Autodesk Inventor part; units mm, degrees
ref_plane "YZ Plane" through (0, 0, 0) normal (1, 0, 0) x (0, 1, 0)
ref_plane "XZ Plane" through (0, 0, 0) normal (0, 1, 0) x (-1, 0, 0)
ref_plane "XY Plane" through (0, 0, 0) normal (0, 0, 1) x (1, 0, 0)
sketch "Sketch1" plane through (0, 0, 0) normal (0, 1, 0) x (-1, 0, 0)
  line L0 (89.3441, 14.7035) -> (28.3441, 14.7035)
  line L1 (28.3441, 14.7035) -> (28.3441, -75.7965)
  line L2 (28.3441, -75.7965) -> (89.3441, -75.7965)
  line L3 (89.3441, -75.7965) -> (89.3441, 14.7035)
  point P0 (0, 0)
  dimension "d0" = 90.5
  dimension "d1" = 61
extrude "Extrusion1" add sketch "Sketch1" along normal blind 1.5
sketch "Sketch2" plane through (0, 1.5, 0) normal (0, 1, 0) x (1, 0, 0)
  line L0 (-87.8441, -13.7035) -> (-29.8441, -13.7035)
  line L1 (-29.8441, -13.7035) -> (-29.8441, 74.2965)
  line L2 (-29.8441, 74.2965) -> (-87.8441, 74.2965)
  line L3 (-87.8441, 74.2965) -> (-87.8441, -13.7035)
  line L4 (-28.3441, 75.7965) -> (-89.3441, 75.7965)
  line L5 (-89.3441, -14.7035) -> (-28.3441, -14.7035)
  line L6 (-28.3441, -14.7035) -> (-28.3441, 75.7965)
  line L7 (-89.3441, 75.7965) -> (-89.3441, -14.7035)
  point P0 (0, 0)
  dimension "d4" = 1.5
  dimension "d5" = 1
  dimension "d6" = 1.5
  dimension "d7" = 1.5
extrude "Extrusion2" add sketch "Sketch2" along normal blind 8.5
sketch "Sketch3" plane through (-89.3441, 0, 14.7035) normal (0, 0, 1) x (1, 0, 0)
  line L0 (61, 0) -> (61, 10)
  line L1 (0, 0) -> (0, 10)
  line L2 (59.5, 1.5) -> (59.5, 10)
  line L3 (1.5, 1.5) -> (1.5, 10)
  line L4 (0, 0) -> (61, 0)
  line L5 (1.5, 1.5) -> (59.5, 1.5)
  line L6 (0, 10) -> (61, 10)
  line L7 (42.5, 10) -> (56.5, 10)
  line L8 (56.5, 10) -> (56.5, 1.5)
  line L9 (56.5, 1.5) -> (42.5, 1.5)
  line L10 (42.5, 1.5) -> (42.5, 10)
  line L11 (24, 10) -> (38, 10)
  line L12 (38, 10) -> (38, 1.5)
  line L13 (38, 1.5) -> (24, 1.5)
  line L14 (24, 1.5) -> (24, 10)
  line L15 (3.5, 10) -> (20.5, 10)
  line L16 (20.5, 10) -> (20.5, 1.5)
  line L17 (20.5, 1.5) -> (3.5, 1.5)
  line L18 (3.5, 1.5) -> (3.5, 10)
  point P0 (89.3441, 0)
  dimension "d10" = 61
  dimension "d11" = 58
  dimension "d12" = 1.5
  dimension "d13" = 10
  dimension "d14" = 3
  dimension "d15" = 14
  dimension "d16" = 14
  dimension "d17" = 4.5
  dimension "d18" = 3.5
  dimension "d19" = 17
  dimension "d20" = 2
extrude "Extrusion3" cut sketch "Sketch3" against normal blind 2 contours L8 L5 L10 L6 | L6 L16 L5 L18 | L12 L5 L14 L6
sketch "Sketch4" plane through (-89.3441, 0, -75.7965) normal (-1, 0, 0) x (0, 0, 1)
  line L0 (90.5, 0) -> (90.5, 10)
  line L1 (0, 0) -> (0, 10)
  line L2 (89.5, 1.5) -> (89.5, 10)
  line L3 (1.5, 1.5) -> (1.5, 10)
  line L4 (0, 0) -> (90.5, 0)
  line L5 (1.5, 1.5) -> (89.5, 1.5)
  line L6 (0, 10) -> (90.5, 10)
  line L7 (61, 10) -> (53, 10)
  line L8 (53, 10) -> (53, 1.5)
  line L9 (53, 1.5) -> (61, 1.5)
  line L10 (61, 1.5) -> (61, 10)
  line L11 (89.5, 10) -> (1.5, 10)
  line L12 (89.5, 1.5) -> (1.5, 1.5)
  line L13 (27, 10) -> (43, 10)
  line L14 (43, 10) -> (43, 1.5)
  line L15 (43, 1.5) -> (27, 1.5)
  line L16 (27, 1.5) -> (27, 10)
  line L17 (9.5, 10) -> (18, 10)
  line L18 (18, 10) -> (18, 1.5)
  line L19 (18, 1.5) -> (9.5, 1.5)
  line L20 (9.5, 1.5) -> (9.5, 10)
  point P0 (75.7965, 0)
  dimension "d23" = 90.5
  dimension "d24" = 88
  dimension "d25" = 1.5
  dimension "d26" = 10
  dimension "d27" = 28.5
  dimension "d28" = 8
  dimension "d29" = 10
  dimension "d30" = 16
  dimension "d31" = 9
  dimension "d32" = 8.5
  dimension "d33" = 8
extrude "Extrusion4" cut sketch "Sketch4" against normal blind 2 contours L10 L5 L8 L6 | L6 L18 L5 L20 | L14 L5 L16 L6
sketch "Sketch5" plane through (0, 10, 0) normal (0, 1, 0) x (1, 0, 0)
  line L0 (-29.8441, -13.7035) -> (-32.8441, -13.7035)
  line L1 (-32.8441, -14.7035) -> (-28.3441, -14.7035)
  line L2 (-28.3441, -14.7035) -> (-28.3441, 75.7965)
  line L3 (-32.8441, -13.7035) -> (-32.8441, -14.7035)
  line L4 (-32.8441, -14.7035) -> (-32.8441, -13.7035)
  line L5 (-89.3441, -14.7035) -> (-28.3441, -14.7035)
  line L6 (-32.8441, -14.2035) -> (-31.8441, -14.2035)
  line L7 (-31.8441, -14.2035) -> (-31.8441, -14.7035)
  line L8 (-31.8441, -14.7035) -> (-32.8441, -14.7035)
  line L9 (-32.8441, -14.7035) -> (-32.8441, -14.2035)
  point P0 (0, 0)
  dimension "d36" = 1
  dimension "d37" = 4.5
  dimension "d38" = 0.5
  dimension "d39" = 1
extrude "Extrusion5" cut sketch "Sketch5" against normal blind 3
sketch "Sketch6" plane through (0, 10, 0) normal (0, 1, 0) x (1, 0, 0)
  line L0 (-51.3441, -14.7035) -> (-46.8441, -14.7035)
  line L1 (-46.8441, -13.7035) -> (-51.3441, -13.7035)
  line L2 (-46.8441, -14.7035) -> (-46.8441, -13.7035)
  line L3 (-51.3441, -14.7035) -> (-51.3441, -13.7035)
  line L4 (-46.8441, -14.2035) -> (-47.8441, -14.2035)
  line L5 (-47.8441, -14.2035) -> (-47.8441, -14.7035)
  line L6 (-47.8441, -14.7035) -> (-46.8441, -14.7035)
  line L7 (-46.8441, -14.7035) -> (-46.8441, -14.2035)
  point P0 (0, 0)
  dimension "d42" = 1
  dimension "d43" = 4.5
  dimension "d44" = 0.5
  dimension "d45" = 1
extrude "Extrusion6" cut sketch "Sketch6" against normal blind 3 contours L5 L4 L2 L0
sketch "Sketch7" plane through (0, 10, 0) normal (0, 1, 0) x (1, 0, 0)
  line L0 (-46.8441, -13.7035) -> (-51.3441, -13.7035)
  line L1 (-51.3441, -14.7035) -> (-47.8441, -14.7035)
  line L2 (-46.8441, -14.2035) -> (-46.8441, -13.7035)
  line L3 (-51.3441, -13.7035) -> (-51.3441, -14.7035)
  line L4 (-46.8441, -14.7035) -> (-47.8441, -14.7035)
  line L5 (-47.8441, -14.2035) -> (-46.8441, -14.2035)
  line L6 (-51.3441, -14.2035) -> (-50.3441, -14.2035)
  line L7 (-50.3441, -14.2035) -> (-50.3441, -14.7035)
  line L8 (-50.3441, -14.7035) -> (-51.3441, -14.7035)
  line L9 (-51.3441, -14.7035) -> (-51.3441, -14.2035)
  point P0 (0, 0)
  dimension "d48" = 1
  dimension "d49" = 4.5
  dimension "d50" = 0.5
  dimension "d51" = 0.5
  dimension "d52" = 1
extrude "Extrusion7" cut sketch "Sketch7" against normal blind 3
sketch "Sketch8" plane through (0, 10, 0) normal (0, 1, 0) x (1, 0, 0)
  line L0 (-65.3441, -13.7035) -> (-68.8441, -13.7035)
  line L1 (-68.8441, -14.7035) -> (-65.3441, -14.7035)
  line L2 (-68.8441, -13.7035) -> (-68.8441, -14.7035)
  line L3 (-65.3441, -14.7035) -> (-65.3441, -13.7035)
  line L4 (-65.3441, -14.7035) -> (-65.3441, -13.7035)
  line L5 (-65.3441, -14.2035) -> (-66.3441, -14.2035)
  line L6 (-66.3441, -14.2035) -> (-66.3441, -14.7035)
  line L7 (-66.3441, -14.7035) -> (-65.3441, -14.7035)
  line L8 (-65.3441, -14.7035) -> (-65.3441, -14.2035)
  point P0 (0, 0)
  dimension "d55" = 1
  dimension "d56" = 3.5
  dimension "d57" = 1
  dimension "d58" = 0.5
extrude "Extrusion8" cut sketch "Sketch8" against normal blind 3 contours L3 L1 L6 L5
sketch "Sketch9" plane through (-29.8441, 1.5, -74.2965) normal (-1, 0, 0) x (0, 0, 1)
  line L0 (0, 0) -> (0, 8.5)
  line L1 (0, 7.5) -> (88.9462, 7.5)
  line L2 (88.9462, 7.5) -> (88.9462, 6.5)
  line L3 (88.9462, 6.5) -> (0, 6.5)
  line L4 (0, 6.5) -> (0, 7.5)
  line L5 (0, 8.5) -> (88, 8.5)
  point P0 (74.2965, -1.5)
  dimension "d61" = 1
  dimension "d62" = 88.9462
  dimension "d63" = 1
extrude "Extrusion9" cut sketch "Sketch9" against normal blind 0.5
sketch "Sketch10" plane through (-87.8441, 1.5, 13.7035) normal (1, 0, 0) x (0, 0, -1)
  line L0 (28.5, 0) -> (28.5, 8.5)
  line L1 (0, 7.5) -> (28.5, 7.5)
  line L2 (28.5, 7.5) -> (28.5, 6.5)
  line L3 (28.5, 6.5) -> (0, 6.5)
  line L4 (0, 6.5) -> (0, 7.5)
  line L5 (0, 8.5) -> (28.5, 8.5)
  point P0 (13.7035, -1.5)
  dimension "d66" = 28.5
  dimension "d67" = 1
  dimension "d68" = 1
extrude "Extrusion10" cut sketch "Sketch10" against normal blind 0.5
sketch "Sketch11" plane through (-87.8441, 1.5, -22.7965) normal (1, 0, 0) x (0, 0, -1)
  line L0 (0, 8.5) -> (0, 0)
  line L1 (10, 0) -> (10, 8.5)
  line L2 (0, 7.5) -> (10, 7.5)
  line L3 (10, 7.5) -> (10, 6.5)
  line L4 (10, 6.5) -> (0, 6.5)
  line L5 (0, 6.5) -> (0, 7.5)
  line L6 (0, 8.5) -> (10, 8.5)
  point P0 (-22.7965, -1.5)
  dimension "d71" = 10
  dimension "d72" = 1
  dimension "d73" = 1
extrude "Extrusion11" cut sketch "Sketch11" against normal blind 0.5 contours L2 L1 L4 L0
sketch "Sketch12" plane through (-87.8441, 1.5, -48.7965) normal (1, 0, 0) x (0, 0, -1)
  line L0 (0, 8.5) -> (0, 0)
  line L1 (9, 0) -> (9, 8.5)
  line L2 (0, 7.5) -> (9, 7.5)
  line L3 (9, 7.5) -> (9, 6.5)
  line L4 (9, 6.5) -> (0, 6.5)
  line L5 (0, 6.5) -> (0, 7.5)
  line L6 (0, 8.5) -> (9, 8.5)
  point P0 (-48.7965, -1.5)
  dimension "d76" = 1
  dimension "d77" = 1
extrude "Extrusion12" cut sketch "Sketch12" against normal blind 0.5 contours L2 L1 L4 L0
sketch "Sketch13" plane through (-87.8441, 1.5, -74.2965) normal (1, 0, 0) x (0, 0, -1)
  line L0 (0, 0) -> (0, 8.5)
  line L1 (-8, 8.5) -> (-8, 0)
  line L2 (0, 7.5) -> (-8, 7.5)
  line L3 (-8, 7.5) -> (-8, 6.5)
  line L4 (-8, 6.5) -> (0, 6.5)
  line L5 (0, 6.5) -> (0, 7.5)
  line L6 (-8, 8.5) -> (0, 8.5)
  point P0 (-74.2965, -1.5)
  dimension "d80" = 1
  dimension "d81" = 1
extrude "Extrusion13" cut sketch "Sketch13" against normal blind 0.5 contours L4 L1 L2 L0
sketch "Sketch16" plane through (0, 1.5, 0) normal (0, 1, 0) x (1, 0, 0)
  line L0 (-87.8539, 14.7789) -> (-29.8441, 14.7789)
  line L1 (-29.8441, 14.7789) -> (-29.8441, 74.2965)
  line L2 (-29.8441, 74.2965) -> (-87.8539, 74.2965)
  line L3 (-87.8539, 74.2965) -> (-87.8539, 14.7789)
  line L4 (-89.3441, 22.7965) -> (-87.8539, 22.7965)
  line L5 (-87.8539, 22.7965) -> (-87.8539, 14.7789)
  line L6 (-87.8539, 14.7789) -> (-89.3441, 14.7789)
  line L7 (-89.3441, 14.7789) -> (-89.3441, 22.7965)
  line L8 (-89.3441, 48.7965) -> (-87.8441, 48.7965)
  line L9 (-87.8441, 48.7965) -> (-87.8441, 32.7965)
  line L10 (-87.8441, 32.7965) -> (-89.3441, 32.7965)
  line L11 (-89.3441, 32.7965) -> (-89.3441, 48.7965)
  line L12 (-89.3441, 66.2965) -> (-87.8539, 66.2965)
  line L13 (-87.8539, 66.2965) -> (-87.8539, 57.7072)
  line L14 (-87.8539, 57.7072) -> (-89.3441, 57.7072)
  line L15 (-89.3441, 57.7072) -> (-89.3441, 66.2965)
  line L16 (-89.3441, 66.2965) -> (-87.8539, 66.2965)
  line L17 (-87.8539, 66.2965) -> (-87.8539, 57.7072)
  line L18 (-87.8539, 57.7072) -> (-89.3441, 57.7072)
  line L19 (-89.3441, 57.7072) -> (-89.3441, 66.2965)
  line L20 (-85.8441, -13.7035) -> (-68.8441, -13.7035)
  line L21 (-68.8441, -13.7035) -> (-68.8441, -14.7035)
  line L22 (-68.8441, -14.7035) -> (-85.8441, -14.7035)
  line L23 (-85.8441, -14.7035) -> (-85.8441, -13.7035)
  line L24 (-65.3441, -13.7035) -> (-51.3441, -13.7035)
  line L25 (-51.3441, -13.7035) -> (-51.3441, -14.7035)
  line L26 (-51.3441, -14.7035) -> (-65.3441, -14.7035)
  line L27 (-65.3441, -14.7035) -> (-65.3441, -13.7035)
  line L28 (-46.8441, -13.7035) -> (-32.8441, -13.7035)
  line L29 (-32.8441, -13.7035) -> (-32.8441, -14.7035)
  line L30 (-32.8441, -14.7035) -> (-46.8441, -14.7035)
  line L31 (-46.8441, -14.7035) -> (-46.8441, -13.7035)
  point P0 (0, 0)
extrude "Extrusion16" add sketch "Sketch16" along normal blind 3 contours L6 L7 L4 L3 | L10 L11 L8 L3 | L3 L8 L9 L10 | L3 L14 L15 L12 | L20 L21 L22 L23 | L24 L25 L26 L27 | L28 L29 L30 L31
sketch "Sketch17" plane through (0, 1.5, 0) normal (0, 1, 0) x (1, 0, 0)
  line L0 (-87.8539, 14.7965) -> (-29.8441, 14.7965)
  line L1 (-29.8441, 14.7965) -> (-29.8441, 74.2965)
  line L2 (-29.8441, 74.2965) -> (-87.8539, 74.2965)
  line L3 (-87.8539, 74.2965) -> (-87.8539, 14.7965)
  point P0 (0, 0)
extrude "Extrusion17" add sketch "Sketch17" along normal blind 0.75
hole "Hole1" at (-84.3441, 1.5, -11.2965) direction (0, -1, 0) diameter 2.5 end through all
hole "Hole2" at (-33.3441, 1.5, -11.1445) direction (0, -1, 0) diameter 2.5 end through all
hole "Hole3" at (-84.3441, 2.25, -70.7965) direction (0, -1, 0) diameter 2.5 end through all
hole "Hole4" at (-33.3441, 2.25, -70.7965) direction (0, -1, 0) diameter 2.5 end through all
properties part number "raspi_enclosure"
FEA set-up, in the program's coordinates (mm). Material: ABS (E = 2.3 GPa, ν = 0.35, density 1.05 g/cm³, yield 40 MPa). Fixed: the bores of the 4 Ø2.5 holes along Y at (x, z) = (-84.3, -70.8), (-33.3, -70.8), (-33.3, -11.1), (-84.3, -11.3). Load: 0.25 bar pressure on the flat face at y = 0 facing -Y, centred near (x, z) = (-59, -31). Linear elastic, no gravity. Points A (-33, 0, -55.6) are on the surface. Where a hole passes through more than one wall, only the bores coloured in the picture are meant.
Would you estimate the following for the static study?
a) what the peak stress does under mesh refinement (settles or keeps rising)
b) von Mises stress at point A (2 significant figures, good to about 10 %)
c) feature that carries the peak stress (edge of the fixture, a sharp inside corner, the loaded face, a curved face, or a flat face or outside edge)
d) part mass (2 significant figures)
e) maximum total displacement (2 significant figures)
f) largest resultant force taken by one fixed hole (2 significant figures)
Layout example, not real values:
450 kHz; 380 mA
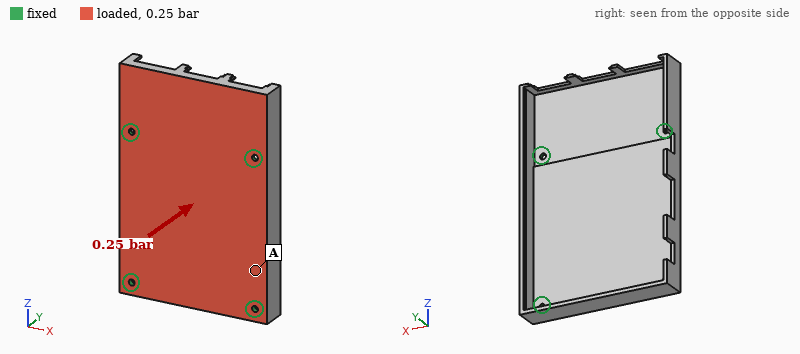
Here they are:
keeps rising; 3.4 MPa; edge of the fixture; 14 g; 1.0 mm; 46 N
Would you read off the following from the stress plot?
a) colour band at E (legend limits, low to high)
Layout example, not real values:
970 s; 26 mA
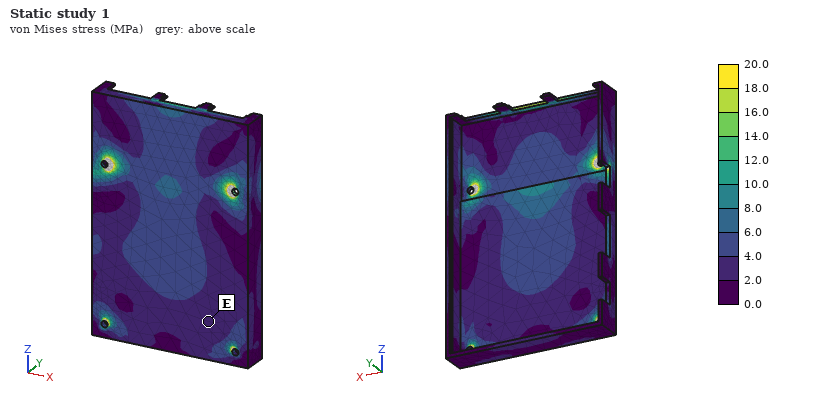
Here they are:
2.0 to 4.0 MPa
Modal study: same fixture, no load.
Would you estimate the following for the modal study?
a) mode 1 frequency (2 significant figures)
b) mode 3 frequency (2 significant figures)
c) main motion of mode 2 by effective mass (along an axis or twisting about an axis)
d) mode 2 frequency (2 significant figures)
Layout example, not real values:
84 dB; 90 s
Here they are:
650 Hz; 1100 Hz; along Y; 750 Hz
